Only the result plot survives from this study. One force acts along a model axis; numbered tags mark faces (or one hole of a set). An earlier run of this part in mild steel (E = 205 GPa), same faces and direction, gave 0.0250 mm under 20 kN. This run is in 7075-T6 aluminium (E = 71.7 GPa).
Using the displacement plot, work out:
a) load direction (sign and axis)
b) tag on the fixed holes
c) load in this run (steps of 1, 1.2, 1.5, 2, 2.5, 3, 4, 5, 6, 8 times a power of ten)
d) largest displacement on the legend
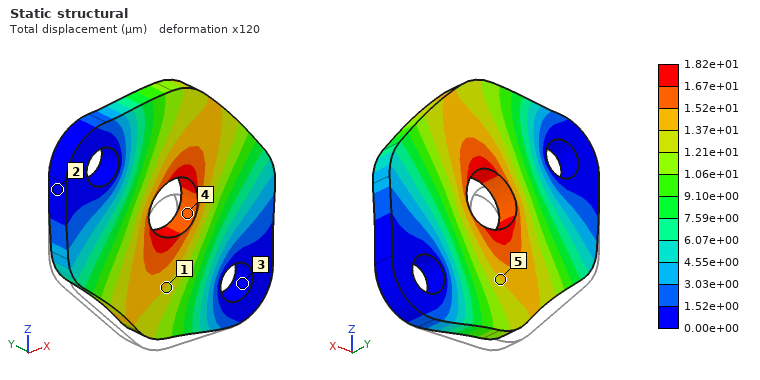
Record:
+Z
3
5 kN
1.82e+01 µm
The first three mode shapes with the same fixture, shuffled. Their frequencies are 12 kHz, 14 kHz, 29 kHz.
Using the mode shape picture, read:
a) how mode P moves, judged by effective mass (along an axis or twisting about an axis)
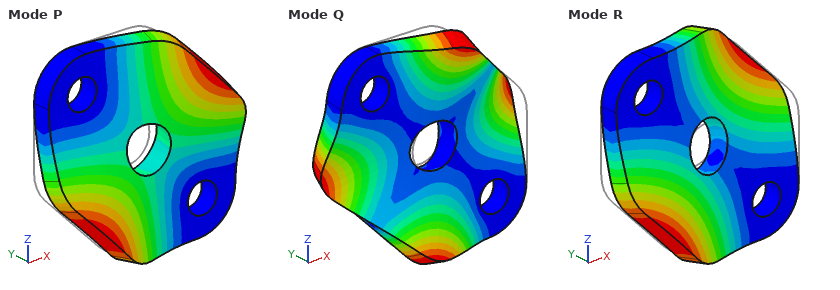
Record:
along Y
